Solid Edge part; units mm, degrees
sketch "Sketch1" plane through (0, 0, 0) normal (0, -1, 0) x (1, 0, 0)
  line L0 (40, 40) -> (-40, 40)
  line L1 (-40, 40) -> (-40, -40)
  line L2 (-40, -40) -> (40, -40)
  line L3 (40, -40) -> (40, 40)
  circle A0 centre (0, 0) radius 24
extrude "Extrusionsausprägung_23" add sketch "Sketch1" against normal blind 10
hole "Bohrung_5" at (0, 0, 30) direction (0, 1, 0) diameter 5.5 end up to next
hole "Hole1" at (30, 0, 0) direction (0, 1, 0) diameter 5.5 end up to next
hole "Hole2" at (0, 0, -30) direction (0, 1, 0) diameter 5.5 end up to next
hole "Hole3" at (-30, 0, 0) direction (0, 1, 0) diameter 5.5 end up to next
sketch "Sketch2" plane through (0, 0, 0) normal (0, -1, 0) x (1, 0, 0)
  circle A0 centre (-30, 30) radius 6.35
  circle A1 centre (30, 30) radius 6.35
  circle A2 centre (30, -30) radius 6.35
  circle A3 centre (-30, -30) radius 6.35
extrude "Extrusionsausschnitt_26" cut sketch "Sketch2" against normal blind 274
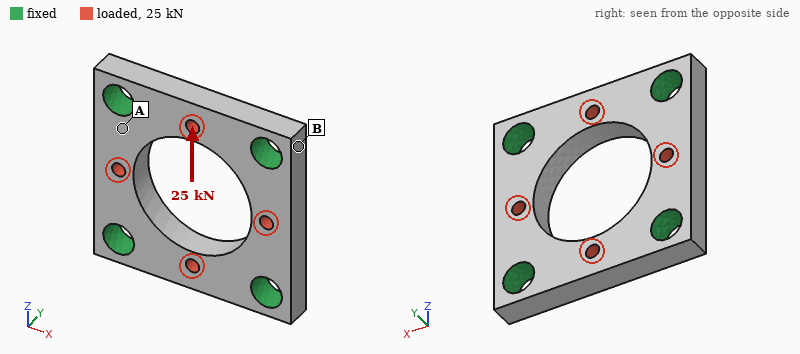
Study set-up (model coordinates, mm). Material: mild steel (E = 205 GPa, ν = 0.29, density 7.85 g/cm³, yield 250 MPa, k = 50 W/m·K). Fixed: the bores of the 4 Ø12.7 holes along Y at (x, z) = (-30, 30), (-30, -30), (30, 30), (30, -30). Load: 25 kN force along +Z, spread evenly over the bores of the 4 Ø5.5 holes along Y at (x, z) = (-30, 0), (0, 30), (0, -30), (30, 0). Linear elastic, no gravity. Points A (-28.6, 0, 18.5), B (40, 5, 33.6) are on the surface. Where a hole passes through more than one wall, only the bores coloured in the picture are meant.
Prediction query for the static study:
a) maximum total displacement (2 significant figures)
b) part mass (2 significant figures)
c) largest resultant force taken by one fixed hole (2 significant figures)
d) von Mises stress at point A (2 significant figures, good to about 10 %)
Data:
11 µm
310 g
6.3 kN
34 MPa
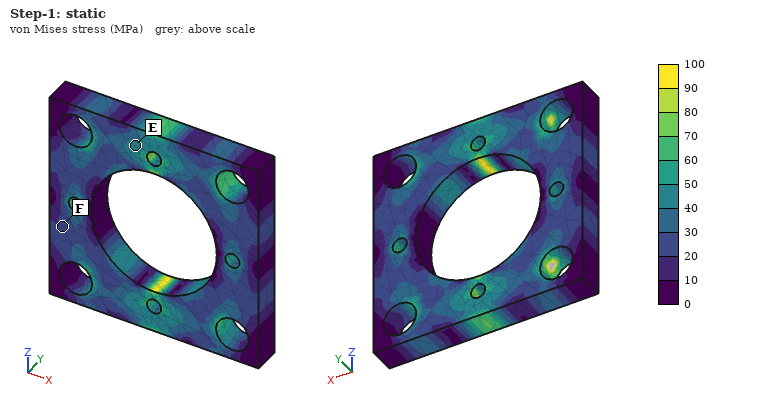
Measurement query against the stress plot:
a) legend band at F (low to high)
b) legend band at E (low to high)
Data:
20 to 30 MPa
40 to 50 MPa
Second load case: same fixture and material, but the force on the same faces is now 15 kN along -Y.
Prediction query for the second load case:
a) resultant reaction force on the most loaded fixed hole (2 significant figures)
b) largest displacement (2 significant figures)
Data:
3.8 kN
13 µm
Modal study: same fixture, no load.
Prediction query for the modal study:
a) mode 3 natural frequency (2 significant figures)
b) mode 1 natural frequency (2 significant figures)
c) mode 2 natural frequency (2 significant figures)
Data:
18 kHz
17 kHz
18 kHz
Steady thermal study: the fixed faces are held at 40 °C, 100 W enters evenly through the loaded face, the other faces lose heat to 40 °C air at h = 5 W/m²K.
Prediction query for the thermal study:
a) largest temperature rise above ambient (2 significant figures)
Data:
37 K
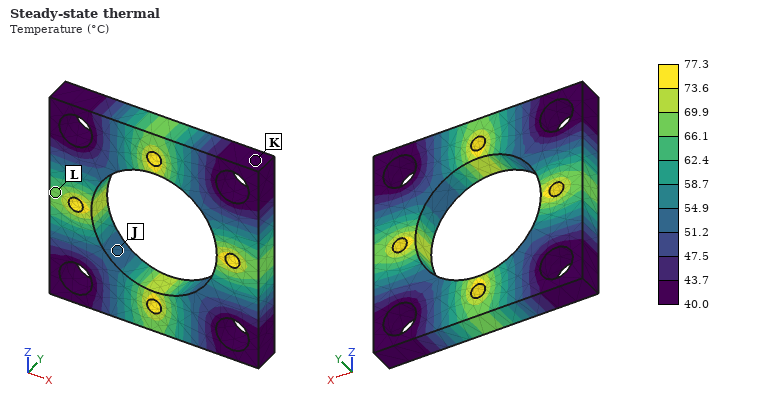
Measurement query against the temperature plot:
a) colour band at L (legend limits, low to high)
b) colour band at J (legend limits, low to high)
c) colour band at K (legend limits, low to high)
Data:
66.1 to 69.9 °C
51.2 to 54.9 °C
40.0 to 43.7 °C
